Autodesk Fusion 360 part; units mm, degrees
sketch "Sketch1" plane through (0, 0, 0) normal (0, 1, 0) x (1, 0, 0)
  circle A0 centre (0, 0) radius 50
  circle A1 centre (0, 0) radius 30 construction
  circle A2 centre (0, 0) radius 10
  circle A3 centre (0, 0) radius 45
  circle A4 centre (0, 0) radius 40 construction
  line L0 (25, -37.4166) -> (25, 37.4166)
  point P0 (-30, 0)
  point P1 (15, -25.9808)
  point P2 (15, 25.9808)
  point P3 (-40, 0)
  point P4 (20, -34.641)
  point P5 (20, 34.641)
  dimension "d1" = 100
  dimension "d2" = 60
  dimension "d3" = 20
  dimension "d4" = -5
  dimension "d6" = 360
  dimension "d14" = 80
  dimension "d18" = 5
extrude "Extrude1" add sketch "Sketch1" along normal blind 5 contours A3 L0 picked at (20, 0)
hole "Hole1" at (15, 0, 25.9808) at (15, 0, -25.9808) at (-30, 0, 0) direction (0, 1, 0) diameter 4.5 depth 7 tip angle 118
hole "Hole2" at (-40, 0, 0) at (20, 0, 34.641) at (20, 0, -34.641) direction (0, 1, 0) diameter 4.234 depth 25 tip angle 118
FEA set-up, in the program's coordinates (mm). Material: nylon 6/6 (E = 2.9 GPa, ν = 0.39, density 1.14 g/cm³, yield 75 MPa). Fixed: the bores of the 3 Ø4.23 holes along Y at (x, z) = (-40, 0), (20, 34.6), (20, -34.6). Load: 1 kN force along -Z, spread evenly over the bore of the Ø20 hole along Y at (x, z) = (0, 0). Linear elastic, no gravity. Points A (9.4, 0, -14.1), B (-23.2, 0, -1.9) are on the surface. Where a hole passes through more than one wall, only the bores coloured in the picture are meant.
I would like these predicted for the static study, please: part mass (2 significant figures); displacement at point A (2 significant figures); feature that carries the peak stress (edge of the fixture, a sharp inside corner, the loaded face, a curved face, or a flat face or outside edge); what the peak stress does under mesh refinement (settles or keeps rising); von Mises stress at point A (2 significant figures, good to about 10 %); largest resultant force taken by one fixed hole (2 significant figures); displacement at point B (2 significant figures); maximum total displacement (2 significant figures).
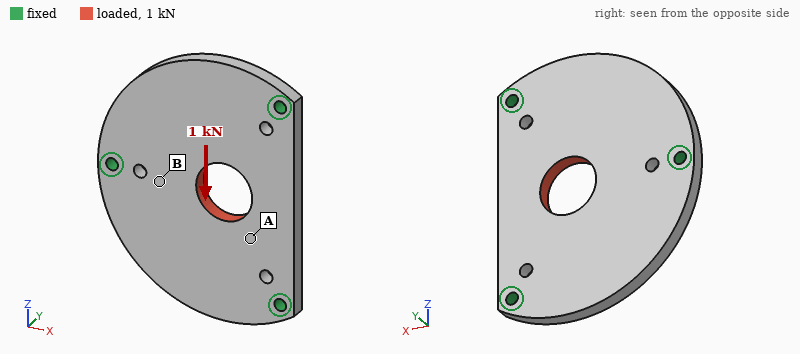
28 g
43 µm
edge of the fixture
keeps rising
2.9 MPa
340 N
38 µm
67 µm
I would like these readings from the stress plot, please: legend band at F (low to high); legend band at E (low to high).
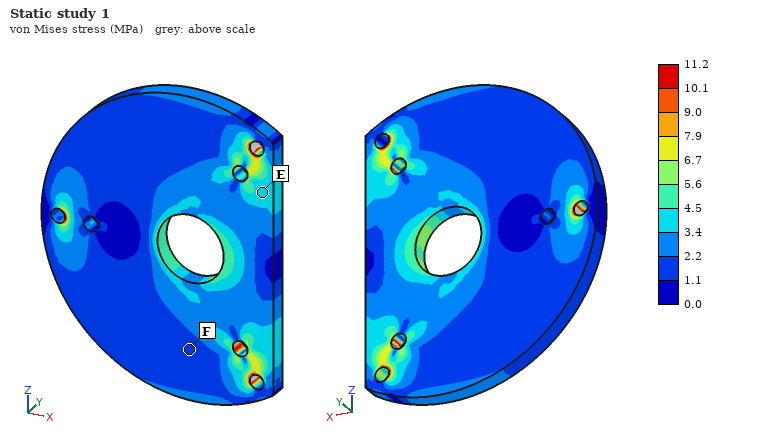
1.1 to 2.2 MPa
3.4 to 4.5 MPa
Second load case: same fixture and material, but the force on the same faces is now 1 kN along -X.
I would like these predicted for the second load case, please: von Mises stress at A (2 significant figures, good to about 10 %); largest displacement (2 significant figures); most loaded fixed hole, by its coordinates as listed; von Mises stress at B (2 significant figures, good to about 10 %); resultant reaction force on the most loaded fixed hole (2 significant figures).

2.9 MPa
97 µm
(-40, 0)
3.9 MPa
400 N
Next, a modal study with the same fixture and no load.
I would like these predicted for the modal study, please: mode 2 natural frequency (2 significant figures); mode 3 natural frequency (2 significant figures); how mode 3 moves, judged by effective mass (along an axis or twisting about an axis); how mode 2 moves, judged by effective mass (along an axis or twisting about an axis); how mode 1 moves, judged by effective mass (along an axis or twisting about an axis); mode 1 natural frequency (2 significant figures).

1200 Hz
1600 Hz
along Y
along Y
twisting about X
1100 Hz
